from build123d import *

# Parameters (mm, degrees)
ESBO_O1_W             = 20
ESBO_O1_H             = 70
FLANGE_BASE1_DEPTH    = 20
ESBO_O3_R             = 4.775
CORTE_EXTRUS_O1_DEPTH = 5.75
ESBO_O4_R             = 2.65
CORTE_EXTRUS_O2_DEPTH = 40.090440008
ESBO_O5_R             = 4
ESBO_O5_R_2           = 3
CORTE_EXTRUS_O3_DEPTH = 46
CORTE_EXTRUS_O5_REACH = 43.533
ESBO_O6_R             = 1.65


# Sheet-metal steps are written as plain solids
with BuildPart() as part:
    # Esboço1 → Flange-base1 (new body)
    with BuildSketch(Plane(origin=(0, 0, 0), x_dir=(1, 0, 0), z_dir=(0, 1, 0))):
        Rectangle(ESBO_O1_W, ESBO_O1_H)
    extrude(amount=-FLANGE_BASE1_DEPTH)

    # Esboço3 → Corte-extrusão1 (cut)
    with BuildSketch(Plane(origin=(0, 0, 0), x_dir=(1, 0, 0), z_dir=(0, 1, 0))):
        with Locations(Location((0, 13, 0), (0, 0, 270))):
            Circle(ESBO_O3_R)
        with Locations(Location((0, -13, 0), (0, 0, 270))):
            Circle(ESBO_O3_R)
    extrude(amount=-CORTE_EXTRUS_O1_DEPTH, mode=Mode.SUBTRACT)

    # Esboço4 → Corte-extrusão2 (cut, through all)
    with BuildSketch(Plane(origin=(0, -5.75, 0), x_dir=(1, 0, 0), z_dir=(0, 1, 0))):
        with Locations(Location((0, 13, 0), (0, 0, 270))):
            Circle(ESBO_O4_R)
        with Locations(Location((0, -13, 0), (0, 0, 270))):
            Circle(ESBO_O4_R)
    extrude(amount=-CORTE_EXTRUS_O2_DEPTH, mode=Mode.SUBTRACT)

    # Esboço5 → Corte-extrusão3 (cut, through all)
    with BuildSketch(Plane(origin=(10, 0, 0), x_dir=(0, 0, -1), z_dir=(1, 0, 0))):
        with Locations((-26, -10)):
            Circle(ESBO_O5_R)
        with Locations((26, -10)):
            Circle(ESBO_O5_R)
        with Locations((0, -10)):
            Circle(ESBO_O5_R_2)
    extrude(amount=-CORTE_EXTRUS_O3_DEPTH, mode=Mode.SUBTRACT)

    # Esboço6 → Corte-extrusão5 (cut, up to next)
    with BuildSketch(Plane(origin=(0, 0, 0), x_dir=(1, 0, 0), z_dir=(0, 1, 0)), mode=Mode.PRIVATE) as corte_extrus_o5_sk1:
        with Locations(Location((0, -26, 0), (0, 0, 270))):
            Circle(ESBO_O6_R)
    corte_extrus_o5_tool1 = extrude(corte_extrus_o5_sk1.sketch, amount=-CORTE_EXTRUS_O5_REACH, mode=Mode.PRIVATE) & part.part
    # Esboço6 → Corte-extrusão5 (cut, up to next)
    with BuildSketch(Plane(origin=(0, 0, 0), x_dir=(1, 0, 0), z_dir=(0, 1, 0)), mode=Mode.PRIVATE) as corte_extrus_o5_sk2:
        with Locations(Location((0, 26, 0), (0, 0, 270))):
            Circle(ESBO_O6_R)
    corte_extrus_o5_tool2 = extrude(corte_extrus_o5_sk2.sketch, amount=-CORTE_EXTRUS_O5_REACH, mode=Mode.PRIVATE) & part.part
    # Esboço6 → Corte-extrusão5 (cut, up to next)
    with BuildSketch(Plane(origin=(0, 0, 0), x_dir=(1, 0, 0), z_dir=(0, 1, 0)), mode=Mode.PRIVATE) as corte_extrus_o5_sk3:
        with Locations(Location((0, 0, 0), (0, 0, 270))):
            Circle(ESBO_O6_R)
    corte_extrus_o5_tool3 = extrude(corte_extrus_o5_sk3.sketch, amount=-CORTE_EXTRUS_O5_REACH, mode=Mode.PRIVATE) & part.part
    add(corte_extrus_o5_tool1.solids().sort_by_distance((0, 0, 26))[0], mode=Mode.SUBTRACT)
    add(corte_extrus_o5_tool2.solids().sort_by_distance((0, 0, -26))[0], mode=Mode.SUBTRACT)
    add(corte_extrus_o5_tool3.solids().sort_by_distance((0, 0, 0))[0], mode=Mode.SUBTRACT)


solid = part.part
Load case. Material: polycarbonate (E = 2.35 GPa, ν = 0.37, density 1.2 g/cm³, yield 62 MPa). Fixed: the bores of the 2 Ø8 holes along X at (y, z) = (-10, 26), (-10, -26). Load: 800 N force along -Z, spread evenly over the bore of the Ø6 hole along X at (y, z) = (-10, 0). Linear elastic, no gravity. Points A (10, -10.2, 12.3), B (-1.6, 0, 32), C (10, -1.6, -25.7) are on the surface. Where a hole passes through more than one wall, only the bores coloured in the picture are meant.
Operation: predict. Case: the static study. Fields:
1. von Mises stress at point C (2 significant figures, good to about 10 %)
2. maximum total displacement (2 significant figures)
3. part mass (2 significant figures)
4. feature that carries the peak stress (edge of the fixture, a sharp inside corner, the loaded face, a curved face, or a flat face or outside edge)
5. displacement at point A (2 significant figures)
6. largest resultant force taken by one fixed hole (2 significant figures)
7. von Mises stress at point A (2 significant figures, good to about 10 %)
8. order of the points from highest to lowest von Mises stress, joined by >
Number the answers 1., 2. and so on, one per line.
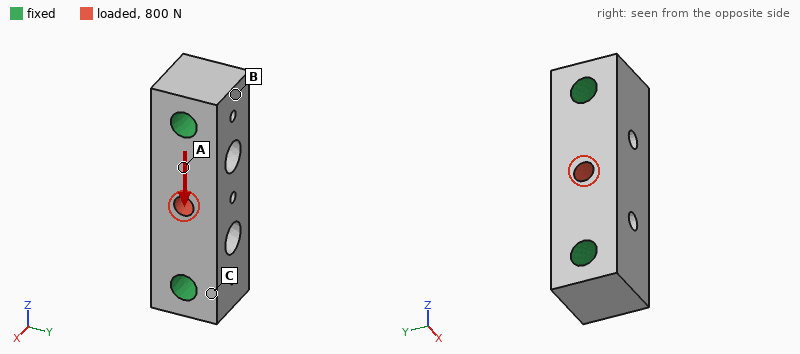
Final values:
1. 0.58 MPa
2. 16 µm
3. 29 g
4. the loaded face
5. 7.6 µm
6. 400 N
7. 1.5 MPa
8. A > C > B
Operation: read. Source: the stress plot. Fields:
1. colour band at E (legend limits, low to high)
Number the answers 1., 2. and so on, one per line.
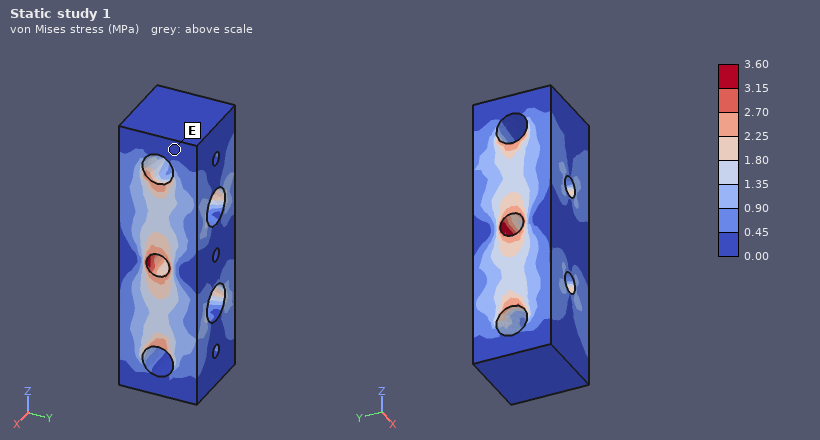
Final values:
1. 0.00 to 0.45 MPa
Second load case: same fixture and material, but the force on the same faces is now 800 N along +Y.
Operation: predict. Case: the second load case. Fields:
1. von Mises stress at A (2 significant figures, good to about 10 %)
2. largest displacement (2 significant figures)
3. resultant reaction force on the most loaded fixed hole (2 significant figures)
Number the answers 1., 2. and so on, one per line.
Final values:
1. 3.2 MPa
2. 65 µm
3. 400 N
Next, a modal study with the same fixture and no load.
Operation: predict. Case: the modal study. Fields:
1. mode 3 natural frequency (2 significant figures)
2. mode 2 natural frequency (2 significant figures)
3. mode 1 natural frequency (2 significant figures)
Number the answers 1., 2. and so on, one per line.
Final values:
1. 7500 Hz
2. 6100 Hz
3. 6000 Hz
